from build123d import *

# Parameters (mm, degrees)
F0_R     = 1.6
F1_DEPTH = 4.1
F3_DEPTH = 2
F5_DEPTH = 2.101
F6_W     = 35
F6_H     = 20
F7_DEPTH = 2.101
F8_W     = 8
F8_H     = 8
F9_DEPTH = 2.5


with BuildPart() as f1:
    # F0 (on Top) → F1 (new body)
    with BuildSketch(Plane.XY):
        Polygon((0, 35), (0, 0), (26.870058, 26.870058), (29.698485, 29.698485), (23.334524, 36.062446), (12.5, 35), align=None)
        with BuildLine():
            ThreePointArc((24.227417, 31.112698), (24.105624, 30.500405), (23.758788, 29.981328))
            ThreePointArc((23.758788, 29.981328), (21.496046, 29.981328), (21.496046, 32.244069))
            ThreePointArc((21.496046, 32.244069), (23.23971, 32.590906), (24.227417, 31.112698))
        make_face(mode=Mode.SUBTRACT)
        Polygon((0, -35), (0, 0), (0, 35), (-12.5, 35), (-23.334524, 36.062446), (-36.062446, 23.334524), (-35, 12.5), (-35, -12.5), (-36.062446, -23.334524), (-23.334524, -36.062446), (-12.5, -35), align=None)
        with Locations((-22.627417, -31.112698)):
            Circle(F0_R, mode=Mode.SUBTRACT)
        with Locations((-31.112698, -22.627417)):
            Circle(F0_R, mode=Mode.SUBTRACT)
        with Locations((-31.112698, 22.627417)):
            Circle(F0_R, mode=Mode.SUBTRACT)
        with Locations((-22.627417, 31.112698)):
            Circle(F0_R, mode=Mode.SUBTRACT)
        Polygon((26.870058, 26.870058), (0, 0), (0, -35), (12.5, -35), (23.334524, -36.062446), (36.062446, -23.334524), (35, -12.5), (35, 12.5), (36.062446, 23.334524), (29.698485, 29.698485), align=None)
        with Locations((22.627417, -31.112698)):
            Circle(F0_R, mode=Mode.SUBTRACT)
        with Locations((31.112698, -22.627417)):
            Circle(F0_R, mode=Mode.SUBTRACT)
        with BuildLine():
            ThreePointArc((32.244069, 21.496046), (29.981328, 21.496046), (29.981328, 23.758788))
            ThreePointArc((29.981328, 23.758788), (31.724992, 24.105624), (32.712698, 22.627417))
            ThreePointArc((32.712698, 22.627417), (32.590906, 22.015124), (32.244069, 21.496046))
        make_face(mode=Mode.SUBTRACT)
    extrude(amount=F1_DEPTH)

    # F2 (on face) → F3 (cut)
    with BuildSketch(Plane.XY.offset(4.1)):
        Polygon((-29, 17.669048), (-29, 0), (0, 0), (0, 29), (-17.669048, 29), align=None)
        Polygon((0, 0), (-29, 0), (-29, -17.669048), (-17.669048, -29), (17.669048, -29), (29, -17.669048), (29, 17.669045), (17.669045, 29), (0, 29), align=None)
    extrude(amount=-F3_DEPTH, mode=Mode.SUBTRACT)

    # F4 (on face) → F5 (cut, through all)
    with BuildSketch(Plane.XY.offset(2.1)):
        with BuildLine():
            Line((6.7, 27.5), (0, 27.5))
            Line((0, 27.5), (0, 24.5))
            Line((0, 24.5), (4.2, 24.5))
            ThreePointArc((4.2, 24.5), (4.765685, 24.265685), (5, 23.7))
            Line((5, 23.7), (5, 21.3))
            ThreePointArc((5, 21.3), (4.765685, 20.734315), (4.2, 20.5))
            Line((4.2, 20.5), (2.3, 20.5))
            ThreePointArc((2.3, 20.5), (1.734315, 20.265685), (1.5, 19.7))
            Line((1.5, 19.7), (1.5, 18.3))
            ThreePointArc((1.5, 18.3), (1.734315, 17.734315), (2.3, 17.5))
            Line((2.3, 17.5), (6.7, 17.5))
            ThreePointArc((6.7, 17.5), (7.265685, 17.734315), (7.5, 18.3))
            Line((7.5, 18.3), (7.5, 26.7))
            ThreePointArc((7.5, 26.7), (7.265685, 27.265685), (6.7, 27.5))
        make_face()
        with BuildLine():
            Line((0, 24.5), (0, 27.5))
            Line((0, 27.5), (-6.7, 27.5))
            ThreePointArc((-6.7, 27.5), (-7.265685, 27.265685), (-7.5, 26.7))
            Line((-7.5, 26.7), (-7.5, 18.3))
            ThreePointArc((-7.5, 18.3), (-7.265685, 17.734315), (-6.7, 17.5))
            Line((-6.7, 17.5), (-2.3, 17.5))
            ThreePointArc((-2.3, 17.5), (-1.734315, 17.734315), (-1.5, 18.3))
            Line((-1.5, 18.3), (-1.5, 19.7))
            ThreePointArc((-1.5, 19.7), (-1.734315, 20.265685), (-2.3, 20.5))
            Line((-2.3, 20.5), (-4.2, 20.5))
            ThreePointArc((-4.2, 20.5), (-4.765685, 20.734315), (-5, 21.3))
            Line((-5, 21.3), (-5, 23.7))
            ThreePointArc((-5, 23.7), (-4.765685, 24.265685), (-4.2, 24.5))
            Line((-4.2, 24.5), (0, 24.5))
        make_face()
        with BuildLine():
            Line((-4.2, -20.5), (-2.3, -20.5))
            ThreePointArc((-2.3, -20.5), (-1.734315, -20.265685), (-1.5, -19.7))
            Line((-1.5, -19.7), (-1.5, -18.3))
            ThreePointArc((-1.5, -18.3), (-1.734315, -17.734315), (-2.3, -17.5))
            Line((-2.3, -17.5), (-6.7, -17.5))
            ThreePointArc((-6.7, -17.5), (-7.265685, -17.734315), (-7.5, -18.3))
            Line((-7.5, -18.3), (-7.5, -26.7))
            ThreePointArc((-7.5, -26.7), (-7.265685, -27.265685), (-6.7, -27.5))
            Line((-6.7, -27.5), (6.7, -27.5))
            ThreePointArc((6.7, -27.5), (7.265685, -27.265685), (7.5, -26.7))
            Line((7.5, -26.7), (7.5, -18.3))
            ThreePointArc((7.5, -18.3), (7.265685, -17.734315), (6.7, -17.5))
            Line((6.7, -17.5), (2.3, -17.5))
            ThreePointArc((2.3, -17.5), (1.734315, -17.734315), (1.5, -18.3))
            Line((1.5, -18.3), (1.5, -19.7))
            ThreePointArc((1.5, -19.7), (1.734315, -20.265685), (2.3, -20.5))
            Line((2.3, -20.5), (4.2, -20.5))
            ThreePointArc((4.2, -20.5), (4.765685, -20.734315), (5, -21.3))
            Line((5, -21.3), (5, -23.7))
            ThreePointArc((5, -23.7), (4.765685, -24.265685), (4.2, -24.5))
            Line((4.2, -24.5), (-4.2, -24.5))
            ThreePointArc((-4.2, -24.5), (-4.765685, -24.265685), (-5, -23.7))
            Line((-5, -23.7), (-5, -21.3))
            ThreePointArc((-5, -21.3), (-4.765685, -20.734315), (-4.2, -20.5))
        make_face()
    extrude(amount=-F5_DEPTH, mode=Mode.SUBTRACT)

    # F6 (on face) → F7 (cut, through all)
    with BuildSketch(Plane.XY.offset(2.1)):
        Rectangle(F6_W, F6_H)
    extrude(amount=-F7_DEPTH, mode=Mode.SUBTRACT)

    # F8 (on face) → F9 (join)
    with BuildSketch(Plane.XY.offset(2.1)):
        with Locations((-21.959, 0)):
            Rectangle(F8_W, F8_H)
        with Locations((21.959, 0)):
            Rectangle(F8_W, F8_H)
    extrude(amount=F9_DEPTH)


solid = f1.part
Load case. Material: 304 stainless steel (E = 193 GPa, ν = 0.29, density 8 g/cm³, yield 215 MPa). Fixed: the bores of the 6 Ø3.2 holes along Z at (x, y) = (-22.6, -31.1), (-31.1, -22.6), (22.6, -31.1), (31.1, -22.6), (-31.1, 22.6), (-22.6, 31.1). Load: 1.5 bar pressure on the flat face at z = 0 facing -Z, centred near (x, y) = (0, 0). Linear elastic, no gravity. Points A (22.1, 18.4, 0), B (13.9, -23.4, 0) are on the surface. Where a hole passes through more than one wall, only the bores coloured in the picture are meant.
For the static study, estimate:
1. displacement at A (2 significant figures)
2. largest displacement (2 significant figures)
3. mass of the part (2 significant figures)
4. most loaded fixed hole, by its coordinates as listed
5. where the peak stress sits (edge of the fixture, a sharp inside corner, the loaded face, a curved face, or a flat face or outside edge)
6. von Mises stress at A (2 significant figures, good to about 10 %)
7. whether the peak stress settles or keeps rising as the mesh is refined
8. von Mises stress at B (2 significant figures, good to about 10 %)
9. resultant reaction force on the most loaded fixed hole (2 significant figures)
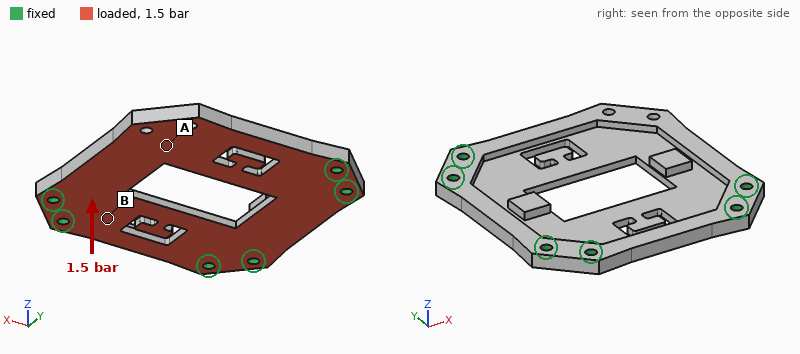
70 µm
98 µm
91 g
(31.1, -22.6)
edge of the fixture
28 MPa
keeps rising
17 MPa
300 N
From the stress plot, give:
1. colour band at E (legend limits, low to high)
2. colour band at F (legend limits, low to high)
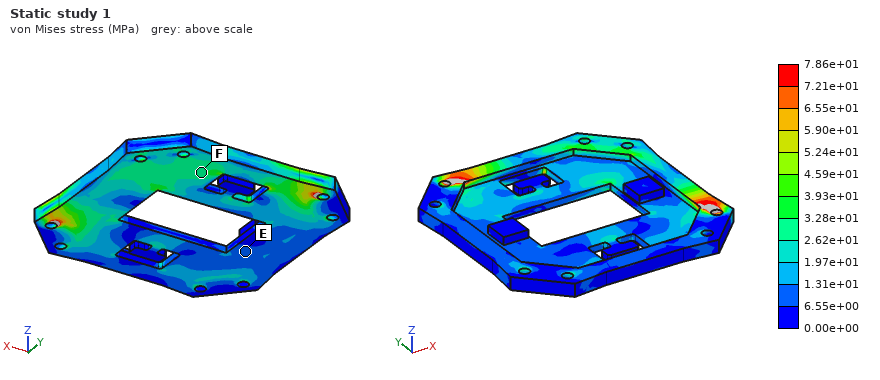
6.55e+00 to 1.31e+01 MPa
2.62e+01 to 3.28e+01 MPa
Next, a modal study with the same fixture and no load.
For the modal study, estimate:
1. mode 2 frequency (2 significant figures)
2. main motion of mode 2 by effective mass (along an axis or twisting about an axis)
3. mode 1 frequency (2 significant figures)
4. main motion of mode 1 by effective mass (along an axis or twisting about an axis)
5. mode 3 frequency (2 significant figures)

4200 Hz
along Z
1500 Hz
along Z
5000 Hz
